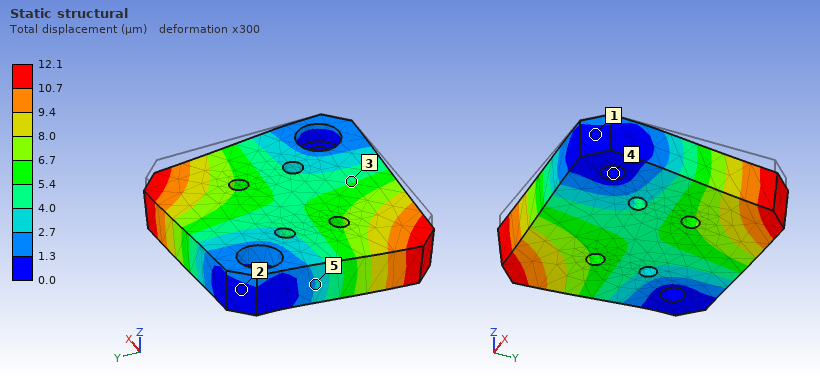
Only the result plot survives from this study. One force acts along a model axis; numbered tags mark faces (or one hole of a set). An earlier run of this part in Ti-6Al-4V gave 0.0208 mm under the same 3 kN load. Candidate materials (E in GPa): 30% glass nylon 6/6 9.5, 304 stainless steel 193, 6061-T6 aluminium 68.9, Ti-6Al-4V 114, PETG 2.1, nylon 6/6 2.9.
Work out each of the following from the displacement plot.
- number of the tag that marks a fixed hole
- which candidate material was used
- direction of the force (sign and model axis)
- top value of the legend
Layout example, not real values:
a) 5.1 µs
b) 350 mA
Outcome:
a) 4
b) 304 stainless steel
c) -Z
d) 12.1 µm
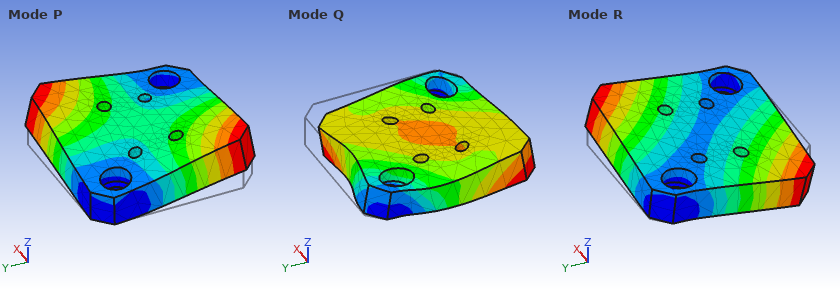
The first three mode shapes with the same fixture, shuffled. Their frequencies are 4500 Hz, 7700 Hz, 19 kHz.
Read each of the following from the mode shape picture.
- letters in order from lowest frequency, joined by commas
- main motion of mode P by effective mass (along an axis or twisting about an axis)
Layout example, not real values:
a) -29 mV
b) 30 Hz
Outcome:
a) R, P, Q
b) along Z
